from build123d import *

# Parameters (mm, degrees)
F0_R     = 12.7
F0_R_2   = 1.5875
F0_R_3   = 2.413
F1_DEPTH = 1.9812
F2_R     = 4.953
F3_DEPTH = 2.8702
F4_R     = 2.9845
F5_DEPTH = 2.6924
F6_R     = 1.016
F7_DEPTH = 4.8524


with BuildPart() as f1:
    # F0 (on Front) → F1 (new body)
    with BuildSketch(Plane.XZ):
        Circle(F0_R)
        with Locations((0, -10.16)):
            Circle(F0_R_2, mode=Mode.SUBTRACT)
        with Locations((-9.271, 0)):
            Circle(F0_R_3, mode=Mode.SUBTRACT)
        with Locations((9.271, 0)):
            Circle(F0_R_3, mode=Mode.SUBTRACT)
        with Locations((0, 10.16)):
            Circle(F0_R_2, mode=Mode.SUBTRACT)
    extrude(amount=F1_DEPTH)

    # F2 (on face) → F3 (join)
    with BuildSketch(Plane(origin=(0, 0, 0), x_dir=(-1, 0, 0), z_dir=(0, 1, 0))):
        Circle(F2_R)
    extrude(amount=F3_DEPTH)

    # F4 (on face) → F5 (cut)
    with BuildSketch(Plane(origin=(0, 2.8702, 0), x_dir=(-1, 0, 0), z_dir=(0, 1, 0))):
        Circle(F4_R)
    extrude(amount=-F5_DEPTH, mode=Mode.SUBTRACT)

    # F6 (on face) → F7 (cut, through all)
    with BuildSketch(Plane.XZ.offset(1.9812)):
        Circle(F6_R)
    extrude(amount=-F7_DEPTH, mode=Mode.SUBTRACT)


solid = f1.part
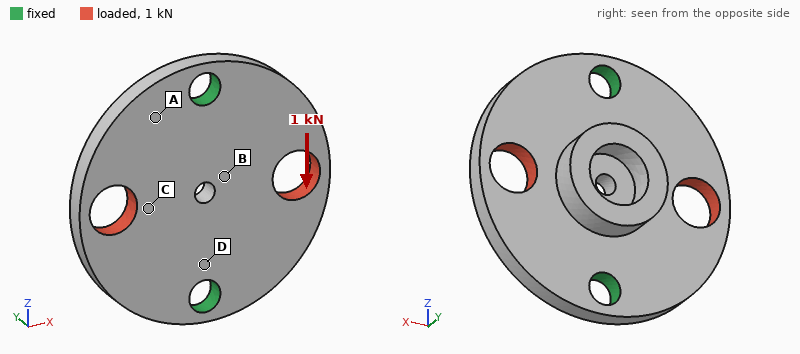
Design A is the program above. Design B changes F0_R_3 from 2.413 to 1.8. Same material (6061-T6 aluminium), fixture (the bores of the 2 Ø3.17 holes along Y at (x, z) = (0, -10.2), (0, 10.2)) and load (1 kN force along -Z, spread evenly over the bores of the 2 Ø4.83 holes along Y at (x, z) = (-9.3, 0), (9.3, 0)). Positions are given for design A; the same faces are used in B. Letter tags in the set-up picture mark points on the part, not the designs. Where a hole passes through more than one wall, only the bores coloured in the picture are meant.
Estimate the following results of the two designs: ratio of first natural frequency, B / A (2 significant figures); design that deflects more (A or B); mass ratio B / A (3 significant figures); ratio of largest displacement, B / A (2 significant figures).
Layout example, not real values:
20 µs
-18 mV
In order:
0.96
A
1.03
0.83
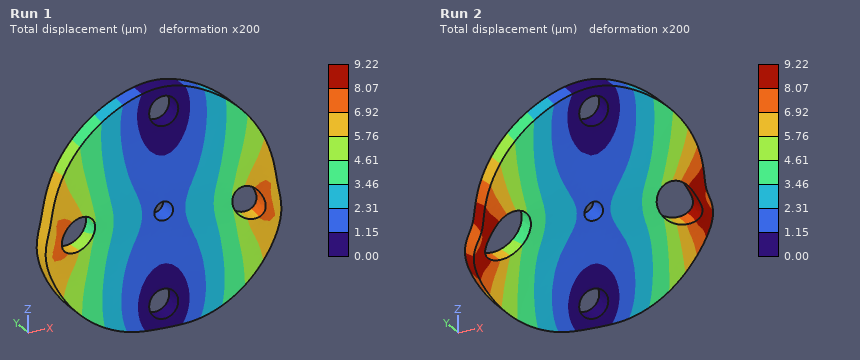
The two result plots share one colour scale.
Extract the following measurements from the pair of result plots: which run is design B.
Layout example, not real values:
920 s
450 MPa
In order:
Run 1
